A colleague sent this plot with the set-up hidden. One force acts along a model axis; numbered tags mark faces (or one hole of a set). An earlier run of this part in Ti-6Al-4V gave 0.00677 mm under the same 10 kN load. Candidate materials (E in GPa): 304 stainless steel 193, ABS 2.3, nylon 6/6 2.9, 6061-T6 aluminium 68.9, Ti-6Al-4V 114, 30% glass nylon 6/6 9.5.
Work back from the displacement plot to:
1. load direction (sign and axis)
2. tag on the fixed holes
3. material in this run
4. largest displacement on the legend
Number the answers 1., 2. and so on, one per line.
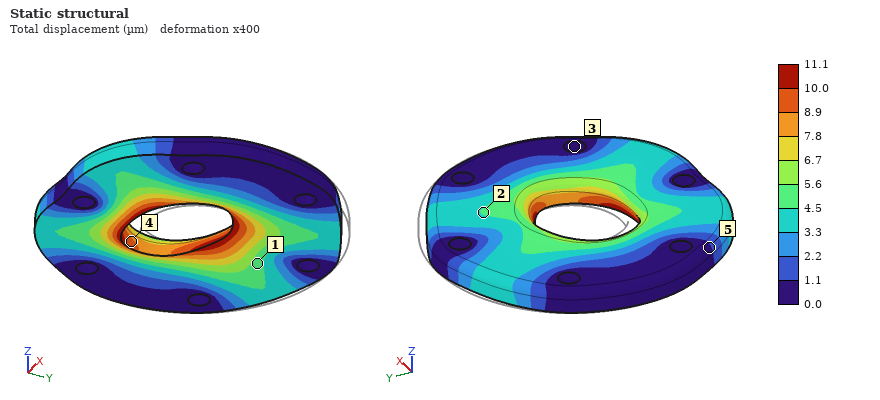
1. -Y
2. 3
3. 6061-T6 aluminium
4. 11.1 µm
